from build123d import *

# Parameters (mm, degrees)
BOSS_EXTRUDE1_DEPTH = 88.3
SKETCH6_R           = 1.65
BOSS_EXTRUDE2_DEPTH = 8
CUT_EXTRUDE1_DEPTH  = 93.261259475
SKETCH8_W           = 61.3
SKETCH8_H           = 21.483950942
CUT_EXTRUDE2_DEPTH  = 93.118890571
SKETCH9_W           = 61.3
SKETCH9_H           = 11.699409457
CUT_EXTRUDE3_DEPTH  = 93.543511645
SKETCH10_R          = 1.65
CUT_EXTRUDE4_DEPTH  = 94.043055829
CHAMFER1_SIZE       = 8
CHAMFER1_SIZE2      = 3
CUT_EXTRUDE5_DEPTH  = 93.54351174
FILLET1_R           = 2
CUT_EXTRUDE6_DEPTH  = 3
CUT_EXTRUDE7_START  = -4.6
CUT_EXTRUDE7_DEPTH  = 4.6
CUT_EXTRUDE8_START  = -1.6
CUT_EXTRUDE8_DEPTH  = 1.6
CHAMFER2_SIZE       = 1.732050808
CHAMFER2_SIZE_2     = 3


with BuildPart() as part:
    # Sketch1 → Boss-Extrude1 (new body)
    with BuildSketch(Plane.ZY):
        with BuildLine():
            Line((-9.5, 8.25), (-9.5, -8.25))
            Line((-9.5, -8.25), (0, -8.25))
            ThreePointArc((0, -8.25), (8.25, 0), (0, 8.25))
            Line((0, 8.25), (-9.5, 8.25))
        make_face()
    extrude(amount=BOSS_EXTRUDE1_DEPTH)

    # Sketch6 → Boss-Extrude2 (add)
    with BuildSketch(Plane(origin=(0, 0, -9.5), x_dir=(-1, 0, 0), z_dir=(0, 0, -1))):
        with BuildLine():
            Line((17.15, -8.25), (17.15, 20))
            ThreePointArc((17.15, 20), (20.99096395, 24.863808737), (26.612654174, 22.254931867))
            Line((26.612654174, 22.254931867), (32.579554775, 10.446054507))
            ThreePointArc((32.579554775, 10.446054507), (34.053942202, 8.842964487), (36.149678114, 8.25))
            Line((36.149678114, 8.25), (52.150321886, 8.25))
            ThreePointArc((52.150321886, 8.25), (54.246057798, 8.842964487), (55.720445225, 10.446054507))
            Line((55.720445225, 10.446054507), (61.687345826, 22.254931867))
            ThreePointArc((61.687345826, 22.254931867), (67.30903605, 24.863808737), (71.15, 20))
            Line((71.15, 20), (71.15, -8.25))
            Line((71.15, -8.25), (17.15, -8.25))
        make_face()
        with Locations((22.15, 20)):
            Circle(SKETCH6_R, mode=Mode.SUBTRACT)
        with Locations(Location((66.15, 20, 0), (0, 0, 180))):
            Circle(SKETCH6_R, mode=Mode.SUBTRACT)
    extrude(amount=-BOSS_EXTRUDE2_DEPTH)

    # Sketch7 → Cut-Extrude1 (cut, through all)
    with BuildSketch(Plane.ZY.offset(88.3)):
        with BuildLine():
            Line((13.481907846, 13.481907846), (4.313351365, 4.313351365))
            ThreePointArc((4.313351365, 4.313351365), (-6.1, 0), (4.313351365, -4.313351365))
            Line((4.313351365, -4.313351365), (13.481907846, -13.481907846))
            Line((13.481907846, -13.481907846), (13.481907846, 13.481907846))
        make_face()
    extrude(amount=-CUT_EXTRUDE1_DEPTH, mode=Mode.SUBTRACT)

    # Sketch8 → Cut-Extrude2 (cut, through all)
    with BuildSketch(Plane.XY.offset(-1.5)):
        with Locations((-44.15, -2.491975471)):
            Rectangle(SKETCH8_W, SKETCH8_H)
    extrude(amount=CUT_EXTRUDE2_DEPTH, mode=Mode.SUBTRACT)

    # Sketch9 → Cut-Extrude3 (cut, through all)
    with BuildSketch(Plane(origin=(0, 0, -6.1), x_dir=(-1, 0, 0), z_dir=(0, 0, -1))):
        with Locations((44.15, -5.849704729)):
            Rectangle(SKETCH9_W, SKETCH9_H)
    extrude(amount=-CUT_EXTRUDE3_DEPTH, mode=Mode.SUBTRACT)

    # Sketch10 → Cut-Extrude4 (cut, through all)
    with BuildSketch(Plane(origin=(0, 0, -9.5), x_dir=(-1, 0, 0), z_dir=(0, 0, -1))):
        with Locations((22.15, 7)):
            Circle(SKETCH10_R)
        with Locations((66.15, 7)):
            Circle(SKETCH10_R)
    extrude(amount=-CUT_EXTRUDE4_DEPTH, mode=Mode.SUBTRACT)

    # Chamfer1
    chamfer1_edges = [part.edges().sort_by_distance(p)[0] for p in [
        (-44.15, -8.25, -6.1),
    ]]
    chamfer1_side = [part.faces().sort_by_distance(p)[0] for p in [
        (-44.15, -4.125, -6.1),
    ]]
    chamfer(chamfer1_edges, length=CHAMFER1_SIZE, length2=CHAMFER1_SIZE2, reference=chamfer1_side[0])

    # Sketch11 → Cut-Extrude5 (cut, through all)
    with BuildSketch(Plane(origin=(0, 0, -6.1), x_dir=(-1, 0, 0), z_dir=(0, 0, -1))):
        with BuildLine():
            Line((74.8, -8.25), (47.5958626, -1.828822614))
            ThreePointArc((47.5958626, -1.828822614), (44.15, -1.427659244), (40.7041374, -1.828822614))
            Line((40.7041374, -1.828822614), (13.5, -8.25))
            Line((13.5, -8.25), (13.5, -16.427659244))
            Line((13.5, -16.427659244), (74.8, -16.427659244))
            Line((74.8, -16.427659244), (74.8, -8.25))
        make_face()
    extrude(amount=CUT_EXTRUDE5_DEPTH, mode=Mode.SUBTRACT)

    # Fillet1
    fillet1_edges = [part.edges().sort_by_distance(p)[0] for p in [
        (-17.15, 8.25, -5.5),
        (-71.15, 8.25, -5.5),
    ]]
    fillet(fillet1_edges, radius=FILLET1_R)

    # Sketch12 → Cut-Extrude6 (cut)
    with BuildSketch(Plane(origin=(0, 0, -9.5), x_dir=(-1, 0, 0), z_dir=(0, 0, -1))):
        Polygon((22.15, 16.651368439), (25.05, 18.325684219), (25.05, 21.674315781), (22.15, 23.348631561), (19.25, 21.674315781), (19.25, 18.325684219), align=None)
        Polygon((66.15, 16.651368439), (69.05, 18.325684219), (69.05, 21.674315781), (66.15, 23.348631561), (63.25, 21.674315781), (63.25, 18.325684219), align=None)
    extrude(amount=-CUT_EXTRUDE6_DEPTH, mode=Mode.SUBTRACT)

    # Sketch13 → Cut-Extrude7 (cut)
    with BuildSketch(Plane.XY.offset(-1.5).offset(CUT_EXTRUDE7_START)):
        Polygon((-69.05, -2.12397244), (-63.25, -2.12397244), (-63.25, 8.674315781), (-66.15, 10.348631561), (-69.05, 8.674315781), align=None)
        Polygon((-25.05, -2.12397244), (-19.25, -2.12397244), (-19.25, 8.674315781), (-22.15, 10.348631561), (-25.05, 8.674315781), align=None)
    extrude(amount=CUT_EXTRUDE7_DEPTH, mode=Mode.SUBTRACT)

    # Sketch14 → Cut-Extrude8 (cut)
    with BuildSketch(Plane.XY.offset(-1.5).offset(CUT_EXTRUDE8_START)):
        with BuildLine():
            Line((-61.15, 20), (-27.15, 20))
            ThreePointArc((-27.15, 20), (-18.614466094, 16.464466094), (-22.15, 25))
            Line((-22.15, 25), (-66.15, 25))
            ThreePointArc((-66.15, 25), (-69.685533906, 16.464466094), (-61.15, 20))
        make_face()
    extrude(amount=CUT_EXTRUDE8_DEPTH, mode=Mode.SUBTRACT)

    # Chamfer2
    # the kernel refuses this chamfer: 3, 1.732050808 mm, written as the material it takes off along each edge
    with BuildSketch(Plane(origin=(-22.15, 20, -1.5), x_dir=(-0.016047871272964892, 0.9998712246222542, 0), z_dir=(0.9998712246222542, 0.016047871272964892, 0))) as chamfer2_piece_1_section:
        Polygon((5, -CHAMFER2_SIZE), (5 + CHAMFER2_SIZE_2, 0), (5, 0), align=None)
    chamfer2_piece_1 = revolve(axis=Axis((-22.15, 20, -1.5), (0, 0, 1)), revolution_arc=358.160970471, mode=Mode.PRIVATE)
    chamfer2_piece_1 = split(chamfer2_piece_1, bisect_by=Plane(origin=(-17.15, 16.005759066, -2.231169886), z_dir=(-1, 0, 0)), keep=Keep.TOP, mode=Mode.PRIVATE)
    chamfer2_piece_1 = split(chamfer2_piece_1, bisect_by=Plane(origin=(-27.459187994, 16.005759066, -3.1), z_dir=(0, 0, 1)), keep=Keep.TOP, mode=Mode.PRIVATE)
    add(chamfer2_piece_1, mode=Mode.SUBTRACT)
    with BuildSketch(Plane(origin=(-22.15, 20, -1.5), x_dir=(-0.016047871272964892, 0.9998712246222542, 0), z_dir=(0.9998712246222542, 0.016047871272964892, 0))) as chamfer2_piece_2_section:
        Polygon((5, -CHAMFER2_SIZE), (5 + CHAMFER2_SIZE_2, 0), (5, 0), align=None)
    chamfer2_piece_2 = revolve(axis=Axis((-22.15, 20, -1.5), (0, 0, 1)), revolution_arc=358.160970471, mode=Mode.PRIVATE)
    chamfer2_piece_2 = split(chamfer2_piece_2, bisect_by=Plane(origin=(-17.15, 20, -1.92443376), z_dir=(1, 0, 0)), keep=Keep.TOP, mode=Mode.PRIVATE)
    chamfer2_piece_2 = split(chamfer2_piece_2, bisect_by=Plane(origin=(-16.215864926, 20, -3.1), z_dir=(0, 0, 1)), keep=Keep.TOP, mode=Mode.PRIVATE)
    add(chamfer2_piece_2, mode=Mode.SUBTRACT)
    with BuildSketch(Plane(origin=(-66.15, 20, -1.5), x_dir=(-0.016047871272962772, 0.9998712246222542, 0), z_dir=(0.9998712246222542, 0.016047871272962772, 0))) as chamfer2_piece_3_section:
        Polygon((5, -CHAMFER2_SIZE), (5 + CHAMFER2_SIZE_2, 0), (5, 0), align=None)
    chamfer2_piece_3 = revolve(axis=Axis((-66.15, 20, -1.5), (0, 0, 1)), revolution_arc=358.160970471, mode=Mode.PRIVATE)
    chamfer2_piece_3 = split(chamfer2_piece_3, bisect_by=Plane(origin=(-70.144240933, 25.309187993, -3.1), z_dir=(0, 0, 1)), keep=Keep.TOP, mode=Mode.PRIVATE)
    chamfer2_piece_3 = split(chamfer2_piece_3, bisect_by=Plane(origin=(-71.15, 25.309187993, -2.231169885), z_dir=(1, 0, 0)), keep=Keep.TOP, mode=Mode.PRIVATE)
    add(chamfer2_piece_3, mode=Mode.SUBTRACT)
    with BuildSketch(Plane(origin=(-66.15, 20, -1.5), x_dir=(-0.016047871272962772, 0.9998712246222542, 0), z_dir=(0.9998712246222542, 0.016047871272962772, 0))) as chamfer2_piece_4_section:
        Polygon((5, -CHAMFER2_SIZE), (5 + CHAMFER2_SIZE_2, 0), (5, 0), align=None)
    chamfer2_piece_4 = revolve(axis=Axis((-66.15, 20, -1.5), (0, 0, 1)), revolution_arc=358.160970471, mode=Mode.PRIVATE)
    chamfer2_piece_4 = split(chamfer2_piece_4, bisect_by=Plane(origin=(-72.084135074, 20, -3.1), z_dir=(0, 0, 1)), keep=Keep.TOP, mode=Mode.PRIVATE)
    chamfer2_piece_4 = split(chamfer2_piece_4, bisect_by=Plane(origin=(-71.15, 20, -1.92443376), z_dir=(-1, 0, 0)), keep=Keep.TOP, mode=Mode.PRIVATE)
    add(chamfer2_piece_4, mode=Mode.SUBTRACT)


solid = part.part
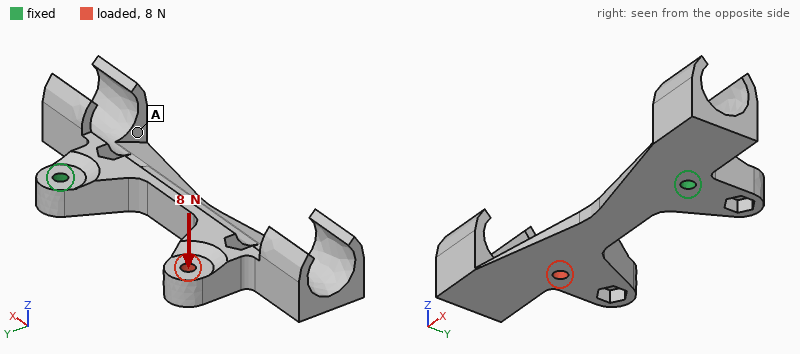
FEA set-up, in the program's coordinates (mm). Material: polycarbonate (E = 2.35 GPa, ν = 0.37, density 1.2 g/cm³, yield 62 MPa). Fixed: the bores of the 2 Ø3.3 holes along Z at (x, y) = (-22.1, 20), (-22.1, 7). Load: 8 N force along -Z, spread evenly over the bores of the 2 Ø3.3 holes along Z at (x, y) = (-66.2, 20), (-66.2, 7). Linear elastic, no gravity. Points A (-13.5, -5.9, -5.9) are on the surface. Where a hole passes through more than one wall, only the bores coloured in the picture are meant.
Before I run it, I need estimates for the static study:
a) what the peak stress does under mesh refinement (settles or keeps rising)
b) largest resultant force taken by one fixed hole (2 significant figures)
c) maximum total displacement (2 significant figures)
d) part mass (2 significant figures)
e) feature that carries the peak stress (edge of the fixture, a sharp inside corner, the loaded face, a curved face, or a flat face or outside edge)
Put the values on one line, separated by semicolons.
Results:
keeps rising; 8.7 N; 1.0 mm; 11 g; edge of the fixture
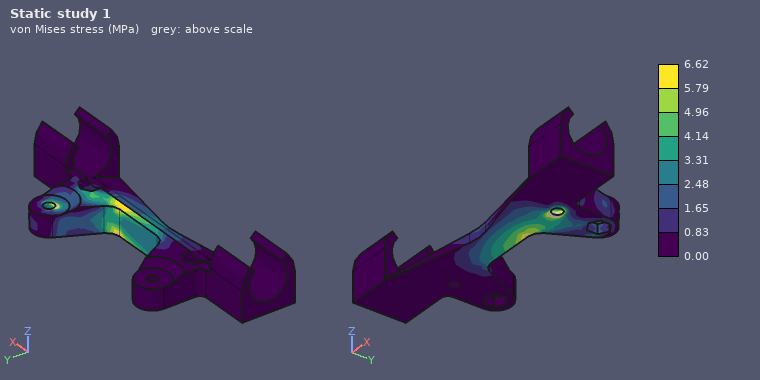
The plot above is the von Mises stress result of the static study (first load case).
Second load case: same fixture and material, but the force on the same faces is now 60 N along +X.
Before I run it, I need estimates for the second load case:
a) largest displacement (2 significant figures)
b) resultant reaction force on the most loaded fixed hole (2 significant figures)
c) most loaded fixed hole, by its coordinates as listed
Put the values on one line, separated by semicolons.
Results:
1.0 mm; 35 N; (-22.1, 7)
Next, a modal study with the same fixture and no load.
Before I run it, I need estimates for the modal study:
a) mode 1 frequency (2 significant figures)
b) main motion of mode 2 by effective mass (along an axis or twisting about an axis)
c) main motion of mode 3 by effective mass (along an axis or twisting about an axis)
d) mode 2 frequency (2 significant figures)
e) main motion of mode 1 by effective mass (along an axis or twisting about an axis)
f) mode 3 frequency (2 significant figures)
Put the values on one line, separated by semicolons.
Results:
210 Hz; along Y; twisting about X; 410 Hz; along Z; 690 Hz
